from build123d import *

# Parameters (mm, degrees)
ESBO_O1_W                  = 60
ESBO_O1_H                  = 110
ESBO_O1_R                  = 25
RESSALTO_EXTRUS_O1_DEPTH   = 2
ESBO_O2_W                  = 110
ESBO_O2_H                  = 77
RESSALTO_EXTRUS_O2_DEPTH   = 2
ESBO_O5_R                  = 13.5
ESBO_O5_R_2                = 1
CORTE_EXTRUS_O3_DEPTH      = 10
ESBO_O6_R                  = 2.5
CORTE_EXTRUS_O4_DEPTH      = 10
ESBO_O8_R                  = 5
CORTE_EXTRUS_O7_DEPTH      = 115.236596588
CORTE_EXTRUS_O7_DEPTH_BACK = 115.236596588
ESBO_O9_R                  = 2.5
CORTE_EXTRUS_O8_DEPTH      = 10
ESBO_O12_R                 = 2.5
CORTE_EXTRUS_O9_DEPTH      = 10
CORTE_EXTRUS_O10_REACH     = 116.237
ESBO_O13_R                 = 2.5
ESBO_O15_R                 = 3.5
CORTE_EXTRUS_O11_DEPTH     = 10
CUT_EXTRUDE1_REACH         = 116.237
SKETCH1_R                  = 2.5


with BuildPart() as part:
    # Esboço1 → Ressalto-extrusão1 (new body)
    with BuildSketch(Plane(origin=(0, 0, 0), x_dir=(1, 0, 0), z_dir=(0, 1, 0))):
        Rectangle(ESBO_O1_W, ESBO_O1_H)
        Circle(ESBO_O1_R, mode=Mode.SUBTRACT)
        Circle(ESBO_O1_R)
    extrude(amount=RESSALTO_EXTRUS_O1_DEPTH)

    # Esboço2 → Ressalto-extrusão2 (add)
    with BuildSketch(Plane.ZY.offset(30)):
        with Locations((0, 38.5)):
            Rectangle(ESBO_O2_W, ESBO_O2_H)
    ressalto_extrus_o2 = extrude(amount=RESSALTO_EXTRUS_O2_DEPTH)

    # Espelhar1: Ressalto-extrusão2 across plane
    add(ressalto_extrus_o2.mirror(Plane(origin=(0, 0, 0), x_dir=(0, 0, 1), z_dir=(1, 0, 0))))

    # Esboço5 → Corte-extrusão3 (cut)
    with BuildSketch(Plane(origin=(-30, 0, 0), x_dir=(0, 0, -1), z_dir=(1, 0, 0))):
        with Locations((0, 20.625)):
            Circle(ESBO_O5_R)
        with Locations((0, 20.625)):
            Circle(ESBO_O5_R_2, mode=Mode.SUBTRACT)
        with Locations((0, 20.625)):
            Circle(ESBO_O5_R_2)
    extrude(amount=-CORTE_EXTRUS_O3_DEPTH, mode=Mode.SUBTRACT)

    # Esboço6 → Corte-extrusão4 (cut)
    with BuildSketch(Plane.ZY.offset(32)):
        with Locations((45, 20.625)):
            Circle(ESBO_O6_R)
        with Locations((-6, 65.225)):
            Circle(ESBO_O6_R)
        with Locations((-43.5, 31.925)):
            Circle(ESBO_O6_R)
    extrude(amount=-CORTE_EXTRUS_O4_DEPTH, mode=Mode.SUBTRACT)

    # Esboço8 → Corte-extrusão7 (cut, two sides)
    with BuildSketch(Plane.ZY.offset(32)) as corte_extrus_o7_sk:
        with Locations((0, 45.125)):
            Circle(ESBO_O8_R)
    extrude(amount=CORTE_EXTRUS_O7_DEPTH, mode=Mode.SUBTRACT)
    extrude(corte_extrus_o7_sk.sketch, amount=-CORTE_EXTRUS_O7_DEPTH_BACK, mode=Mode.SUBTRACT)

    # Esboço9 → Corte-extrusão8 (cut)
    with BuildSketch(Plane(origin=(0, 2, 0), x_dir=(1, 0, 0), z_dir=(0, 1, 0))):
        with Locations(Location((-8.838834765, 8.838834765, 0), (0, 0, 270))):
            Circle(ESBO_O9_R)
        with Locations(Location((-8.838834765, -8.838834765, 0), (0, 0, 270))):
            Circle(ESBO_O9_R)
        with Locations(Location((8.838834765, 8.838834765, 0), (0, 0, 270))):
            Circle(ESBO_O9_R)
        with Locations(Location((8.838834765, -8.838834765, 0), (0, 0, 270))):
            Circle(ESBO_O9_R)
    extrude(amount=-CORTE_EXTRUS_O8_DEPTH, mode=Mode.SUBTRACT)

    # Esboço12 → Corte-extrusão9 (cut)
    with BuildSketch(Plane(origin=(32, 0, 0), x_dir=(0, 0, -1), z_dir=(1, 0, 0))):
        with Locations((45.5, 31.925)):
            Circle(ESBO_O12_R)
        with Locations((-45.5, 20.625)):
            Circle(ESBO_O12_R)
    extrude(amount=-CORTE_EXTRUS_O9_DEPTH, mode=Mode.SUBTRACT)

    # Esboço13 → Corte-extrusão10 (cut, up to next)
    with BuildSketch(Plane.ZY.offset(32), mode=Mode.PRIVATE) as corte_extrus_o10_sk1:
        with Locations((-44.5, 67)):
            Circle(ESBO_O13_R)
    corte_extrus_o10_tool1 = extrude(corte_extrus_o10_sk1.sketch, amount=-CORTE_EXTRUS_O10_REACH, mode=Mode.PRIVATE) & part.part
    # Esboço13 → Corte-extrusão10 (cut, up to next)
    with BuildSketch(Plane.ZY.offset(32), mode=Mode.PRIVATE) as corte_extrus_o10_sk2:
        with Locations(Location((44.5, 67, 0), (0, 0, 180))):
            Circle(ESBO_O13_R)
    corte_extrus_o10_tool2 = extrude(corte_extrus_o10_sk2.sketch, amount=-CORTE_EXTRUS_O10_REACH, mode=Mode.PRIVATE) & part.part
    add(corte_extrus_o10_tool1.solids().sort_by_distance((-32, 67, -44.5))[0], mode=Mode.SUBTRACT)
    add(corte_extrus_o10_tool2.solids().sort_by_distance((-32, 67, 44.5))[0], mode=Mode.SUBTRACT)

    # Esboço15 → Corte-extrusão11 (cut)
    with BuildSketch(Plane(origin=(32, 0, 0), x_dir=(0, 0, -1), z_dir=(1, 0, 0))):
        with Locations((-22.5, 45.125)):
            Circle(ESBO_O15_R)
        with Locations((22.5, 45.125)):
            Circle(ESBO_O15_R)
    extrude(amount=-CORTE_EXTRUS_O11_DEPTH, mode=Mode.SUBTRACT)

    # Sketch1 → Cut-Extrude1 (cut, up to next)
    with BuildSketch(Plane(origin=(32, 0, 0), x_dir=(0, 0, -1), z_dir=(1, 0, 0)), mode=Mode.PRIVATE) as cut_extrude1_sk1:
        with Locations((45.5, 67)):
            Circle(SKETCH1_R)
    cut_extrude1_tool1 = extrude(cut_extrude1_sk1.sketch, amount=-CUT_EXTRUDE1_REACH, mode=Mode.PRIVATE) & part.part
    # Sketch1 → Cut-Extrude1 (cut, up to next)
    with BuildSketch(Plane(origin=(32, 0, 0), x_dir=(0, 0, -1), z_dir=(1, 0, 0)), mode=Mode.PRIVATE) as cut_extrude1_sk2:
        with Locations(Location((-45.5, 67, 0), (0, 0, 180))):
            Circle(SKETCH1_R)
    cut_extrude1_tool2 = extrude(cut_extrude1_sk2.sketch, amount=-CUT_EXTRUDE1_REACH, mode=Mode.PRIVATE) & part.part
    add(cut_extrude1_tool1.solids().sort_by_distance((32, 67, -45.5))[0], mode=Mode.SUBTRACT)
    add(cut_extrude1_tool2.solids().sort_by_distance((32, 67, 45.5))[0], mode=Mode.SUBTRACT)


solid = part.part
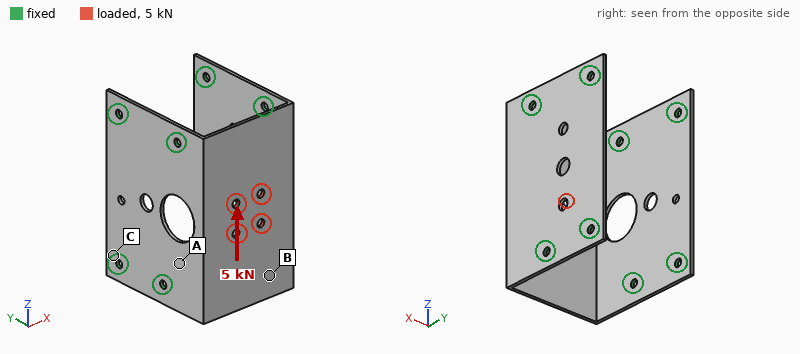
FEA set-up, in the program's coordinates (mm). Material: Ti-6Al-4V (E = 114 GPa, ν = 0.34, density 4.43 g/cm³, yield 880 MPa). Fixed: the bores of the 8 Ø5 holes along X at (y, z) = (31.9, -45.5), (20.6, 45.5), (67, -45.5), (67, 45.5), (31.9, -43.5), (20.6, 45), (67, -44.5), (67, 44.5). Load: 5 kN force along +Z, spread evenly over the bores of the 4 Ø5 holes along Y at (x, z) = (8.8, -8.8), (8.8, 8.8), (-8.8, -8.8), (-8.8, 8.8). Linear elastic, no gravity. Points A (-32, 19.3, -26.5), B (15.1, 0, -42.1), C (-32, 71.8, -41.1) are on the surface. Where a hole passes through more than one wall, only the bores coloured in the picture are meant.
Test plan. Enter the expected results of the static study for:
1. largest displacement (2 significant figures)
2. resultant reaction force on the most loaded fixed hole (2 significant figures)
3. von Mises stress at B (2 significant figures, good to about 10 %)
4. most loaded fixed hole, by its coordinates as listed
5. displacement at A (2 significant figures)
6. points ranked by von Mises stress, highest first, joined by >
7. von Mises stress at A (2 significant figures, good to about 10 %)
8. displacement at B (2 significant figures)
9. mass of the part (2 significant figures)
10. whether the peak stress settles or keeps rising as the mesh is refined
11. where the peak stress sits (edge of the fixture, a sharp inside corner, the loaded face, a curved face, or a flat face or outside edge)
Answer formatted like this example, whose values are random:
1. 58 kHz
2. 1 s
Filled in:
1. 26 µm
2. 1.6 kN
3. 14 MPa
4. (20.6, 45)
5. 8.1 µm
6. A > B > C
7. 30 MPa
8. 18 µm
9. 200 g
10. keeps rising
11. edge of the fixture
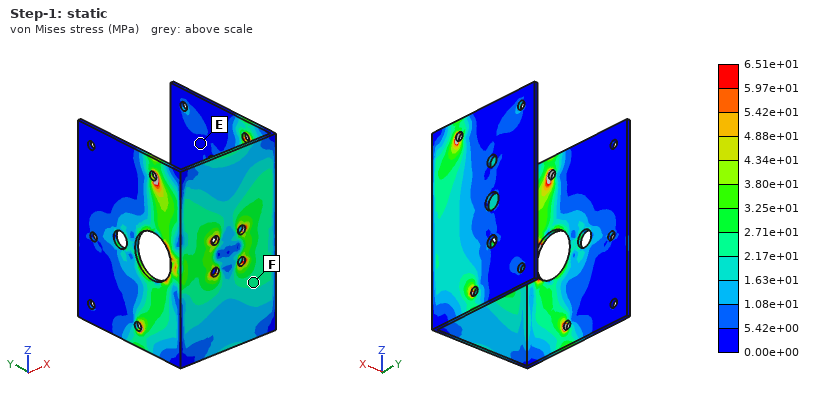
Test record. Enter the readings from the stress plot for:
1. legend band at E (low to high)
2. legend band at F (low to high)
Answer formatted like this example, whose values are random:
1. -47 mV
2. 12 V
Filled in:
1. 0.00e+00 to 5.42e+00 MPa
2. 2.17e+01 to 2.71e+01 MPa
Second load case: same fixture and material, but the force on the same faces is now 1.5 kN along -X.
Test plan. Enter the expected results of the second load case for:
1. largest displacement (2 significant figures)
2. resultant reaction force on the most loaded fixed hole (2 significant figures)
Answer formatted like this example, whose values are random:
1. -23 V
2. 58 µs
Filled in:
1. 0.28 mm
2. 750 N
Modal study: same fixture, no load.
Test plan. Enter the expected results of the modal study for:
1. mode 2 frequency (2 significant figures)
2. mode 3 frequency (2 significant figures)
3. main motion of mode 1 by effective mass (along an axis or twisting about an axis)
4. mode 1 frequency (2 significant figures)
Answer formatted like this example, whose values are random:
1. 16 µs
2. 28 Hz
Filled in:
1. 1400 Hz
2. 1500 Hz
3. along X
4. 1300 Hz
